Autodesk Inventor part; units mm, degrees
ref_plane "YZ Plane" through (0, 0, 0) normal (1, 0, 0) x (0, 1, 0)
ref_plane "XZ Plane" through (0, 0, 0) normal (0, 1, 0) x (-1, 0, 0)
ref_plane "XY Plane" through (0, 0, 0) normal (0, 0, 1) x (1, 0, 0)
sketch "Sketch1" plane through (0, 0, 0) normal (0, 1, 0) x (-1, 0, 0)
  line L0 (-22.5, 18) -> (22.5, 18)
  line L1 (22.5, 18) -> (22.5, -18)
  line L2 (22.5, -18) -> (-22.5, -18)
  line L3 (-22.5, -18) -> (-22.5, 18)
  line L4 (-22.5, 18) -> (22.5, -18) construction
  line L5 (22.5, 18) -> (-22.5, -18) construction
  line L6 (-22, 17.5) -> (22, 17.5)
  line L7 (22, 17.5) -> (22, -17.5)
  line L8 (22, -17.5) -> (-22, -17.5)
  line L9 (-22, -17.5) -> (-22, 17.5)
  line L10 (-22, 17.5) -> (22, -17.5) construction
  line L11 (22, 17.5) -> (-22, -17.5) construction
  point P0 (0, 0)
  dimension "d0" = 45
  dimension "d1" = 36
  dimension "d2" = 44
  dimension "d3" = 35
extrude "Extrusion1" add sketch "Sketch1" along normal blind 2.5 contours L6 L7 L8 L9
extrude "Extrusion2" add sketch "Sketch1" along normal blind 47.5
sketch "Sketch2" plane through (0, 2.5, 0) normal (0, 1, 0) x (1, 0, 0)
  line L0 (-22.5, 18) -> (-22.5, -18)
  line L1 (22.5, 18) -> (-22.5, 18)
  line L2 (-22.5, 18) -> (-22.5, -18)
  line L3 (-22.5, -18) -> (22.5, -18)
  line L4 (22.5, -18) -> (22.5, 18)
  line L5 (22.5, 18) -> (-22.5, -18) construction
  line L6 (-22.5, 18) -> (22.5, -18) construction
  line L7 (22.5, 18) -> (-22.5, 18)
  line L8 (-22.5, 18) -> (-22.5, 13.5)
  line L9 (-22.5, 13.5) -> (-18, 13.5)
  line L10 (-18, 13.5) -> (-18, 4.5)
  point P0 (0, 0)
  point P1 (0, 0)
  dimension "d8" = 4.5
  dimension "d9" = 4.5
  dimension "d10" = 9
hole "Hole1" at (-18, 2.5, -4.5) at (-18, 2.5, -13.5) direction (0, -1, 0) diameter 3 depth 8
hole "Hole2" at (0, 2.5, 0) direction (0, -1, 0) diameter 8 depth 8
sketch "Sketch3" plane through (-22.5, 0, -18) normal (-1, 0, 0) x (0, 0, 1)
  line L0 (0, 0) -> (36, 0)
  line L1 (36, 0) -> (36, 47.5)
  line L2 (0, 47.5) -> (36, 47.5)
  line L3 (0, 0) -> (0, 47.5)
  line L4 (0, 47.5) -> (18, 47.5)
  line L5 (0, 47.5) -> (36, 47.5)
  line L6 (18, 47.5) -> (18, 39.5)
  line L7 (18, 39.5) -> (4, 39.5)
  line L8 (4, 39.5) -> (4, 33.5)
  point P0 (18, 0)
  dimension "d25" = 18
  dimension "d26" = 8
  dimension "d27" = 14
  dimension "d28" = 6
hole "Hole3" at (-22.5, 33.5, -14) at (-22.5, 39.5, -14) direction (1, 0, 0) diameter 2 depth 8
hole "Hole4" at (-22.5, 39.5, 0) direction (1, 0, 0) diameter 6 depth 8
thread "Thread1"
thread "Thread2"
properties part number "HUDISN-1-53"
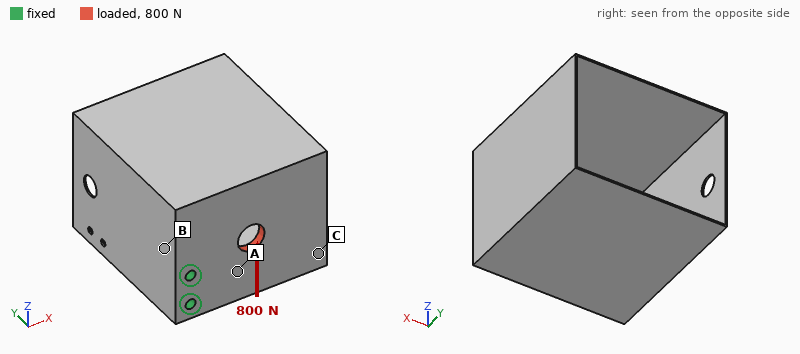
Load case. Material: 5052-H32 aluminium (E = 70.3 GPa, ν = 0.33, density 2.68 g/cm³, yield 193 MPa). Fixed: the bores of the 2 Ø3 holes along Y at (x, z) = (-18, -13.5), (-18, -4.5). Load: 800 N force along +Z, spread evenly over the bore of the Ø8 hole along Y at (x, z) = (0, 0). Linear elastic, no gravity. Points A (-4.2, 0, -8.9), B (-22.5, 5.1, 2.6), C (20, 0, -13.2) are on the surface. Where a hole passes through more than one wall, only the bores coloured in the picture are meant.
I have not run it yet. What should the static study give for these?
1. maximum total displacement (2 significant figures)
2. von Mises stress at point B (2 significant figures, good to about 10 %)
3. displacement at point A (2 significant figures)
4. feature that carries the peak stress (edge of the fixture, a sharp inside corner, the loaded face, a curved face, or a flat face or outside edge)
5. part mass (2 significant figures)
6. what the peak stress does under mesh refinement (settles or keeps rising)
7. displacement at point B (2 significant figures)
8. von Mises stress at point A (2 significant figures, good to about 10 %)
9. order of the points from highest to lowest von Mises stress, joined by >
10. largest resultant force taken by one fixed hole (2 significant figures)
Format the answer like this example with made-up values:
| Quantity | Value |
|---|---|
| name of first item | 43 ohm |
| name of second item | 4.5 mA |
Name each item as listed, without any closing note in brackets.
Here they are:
| Quantity | Value |
|---|---|
| maximum total displacement | 85 µm |
| von Mises stress at point B | 11 MPa |
| displacement at point A | 22 µm |
| feature that carries the peak stress | edge of the fixture |
| part mass | 20 g |
| what the peak stress does under mesh refinement | keeps rising |
| displacement at point B | 14 µm |
| von Mises stress at point A | 26 MPa |
| order of the points from highest to lowest von Mises stress, joined by > | A > B > C |
| largest resultant force taken by one fixed hole | 1.3 kN |
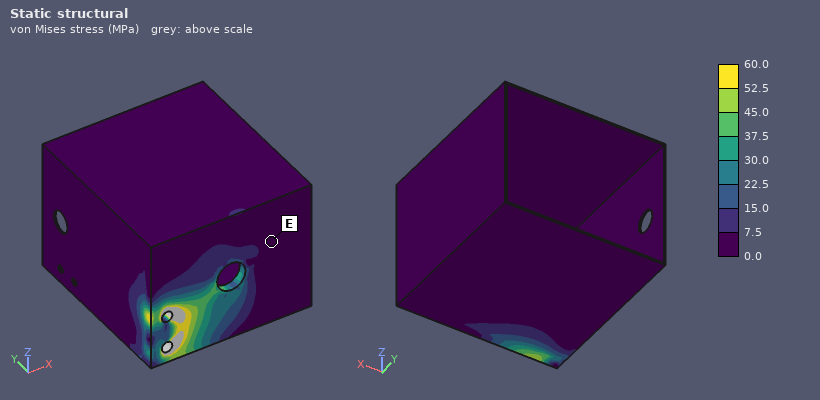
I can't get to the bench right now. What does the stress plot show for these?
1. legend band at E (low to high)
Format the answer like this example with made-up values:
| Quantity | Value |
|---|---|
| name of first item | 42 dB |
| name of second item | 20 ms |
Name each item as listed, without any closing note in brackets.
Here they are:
| Quantity | Value |
|---|---|
| legend band at E | 0.0 to 7.5 MPa |
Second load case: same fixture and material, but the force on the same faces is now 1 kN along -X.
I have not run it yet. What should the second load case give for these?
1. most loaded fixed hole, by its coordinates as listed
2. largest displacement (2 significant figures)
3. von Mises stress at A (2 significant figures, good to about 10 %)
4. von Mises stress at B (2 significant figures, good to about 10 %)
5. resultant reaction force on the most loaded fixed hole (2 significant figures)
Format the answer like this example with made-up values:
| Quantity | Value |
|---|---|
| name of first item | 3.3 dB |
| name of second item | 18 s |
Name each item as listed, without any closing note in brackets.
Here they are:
| Quantity | Value |
|---|---|
| most loaded fixed hole, by its coordinates as listed | (-18, -4.5) |
| largest displacement | 50 µm |
| von Mises stress at A | 15 MPa |
| von Mises stress at B | 7.9 MPa |
| resultant reaction force on the most loaded fixed hole | 1.3 kN |
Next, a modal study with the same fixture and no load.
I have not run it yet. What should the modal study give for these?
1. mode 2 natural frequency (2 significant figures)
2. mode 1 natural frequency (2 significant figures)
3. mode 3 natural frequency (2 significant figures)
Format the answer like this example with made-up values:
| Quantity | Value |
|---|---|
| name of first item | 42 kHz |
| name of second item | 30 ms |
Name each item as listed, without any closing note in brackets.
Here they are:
| Quantity | Value |
|---|---|
| mode 2 natural frequency | 900 Hz |
| mode 1 natural frequency | 690 Hz |
| mode 3 natural frequency | 1100 Hz |
